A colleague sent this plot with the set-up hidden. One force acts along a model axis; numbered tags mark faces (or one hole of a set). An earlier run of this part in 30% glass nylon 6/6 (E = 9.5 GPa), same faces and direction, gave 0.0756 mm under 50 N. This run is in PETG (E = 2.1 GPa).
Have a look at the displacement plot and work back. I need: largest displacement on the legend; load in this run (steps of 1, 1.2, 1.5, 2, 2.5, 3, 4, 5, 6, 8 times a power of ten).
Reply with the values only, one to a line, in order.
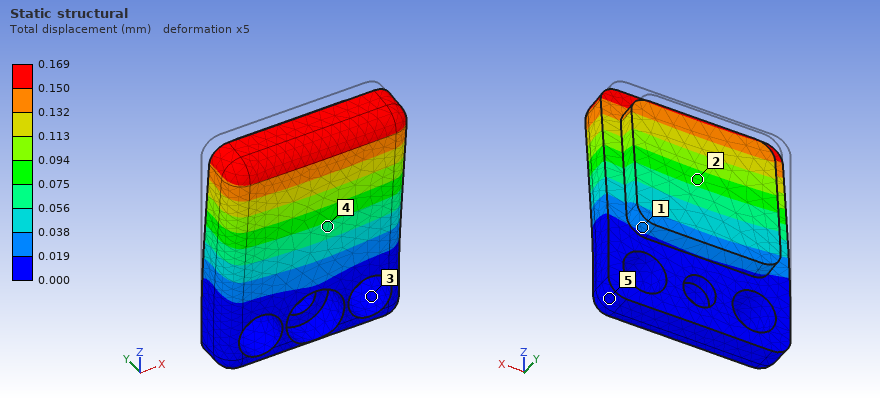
0.169 mm
25 N
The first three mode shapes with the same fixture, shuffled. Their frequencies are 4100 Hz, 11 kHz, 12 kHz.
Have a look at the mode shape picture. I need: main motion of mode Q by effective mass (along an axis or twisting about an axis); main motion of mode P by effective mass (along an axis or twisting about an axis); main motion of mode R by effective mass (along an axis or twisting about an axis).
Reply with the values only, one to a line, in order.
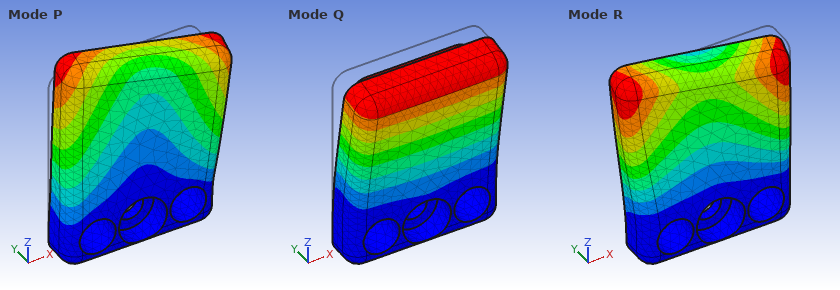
along Y
along X
along X
